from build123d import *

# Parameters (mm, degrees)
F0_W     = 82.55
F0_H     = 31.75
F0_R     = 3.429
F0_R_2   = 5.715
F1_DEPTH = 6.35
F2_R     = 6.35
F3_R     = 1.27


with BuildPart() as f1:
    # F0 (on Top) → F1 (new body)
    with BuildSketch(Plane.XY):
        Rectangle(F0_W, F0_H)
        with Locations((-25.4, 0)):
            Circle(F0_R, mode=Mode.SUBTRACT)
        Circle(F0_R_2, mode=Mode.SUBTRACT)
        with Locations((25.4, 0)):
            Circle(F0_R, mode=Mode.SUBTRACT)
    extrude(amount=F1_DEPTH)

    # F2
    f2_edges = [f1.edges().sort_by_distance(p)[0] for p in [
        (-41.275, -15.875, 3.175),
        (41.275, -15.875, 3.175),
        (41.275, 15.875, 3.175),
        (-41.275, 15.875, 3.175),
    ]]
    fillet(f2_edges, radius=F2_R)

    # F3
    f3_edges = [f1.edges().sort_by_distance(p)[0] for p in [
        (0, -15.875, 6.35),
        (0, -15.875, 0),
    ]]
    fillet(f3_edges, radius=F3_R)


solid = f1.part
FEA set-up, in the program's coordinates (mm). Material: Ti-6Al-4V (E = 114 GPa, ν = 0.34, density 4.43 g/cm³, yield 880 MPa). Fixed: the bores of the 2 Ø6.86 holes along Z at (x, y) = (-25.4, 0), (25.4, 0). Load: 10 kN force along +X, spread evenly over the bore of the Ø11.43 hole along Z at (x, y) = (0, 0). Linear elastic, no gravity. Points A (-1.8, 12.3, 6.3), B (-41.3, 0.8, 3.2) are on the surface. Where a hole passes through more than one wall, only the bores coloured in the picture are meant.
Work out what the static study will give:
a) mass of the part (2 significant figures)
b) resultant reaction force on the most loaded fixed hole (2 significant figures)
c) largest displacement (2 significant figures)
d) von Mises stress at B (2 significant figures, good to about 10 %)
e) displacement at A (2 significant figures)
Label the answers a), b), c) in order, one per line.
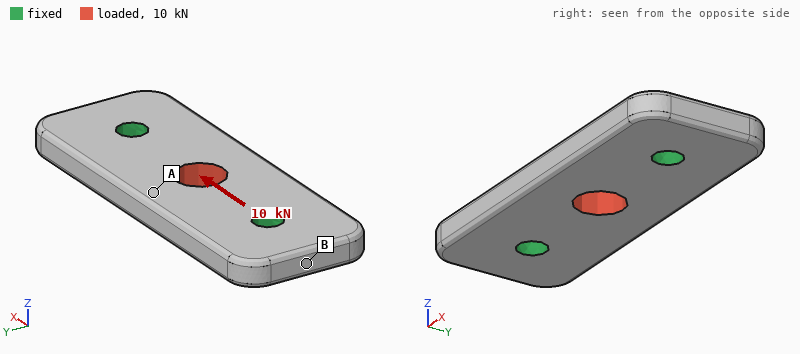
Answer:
a) 67 g
b) 5.0 kN
c) 8.2 µm
d) 15 MPa
e) 4.7 µm
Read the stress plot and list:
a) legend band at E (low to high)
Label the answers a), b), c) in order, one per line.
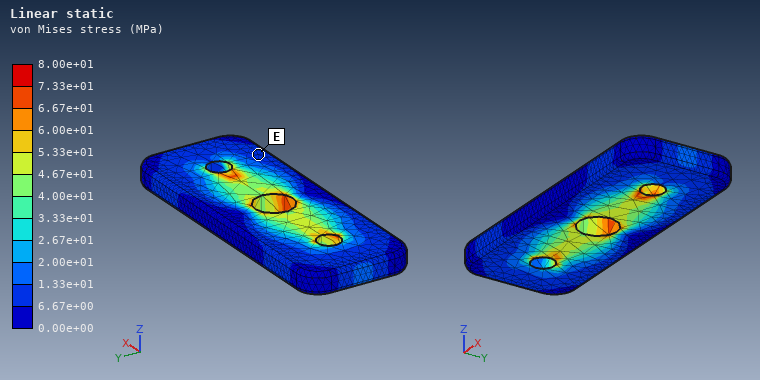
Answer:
a) 6.67e+00 to 1.33e+01 MPa
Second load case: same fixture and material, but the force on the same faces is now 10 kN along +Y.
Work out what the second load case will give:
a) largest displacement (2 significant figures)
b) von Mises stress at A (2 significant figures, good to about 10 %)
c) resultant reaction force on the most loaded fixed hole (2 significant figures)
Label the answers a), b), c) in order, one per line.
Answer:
a) 25 µm
b) 67 MPa
c) 5.0 kN
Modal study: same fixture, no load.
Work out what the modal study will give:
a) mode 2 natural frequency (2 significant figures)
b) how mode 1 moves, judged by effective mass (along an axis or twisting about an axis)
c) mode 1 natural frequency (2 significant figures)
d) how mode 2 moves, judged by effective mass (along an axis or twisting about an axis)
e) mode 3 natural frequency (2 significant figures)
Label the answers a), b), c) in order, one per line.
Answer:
a) 12 kHz
b) along Z
c) 11 kHz
d) twisting about X
e) 19 kHz
